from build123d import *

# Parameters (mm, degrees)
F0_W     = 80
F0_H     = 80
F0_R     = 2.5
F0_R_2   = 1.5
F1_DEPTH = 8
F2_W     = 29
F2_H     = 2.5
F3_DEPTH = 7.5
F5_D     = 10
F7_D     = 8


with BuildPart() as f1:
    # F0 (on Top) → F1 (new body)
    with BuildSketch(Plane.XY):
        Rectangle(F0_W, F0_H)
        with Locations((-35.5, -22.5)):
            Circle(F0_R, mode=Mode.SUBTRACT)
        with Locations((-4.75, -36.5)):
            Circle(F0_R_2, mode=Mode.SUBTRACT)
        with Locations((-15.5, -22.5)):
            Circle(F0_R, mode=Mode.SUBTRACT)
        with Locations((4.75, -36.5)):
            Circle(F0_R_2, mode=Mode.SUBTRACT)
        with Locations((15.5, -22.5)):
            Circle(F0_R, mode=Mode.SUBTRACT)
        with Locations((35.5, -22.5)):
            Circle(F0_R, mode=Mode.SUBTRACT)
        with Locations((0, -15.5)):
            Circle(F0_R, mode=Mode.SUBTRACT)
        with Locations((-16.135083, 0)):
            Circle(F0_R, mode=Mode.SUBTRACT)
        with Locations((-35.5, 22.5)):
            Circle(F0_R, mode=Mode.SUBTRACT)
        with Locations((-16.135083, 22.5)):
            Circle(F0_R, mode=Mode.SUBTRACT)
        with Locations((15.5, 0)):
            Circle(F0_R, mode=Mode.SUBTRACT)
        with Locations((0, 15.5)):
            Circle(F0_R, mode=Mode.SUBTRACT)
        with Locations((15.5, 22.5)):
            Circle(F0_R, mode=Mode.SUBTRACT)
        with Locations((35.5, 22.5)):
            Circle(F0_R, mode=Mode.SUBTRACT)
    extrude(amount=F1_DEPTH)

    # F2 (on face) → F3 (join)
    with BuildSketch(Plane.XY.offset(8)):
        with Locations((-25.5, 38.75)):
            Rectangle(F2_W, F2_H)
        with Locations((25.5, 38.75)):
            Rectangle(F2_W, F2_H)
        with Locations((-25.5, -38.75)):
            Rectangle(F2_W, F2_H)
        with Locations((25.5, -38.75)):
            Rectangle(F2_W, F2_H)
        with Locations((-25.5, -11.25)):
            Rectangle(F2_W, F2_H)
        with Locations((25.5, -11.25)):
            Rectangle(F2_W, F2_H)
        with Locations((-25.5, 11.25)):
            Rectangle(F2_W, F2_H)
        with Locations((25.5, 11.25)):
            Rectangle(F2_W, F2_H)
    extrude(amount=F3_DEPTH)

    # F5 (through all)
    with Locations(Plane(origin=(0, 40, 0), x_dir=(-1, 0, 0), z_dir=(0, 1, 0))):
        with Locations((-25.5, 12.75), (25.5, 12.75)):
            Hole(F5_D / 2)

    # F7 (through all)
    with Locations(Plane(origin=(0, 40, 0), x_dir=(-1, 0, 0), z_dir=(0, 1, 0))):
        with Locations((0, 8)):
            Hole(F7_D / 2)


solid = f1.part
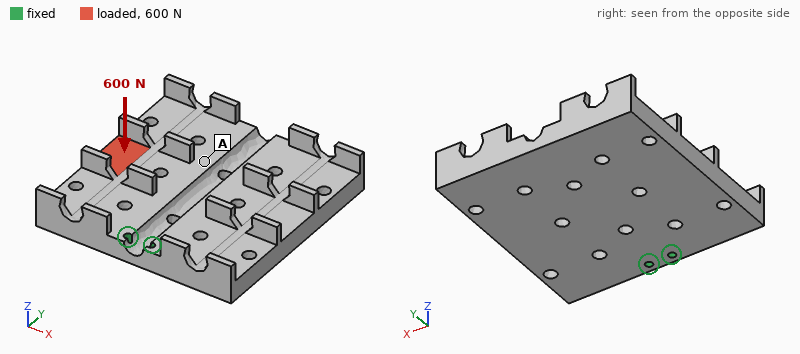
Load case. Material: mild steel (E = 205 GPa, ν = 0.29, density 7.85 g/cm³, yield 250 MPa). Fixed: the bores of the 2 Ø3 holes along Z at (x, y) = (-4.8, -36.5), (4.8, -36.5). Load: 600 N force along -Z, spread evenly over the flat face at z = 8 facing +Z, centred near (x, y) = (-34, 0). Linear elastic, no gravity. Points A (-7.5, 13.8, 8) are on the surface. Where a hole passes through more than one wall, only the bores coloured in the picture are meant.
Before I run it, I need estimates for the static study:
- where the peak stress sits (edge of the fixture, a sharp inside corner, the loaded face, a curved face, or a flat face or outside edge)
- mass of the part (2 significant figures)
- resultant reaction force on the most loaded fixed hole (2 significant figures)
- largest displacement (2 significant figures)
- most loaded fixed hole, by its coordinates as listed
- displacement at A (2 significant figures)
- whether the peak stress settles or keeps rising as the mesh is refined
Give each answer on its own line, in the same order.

edge of the fixture
390 g
1.0 kN
0.16 mm
(-4.8, -36.5)
0.069 mm
keeps rising
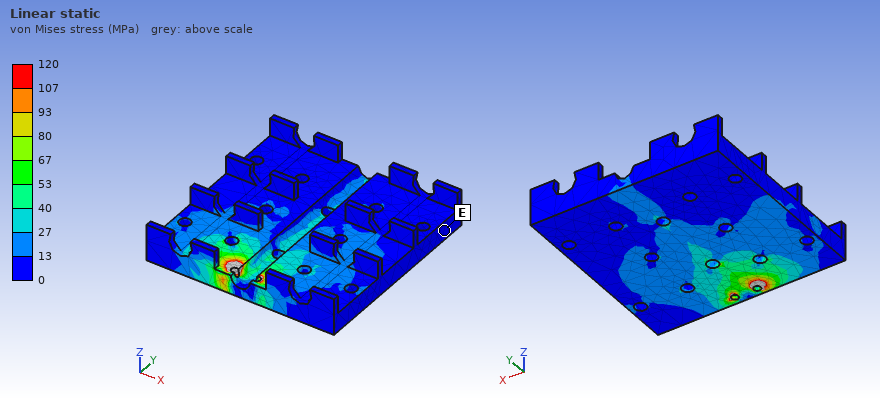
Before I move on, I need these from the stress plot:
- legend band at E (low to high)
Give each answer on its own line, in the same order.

0 to 13 MPa
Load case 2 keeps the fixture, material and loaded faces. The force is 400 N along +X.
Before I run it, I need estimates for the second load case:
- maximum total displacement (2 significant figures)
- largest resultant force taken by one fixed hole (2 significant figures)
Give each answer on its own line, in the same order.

21 µm
1.1 kN
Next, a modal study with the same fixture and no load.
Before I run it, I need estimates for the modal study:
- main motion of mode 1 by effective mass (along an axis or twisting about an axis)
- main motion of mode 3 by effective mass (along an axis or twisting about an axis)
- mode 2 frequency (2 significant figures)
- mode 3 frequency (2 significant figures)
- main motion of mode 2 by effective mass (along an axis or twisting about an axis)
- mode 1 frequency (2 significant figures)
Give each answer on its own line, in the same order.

along Z
along X
1300 Hz
1500 Hz
along X
730 Hz
